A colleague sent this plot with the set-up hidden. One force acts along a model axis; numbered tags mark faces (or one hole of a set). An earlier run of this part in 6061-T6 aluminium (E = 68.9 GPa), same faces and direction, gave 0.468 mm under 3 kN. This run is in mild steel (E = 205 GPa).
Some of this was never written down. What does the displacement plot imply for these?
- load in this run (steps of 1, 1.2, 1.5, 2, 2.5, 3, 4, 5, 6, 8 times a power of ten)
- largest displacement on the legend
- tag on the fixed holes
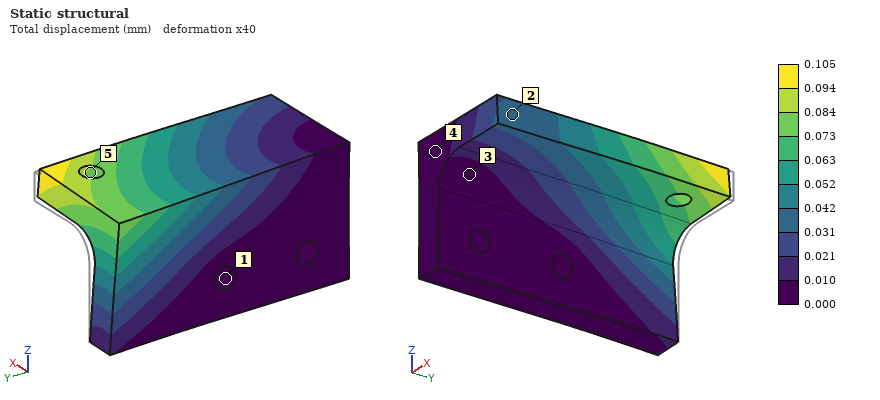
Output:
2 kN
0.105 mm
1
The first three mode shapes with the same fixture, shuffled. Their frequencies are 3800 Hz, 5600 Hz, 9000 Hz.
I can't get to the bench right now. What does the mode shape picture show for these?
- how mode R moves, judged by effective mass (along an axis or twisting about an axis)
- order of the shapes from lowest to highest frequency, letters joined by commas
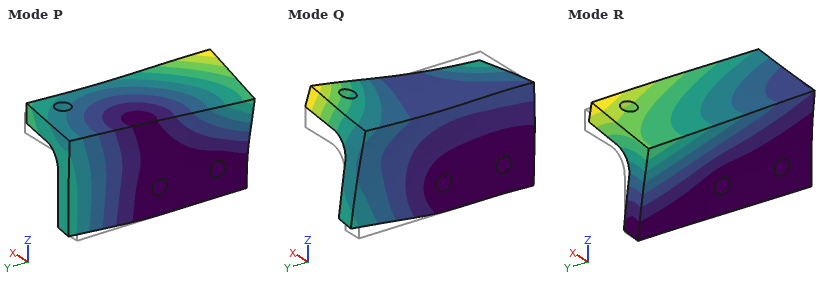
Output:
along X
R, P, Q
